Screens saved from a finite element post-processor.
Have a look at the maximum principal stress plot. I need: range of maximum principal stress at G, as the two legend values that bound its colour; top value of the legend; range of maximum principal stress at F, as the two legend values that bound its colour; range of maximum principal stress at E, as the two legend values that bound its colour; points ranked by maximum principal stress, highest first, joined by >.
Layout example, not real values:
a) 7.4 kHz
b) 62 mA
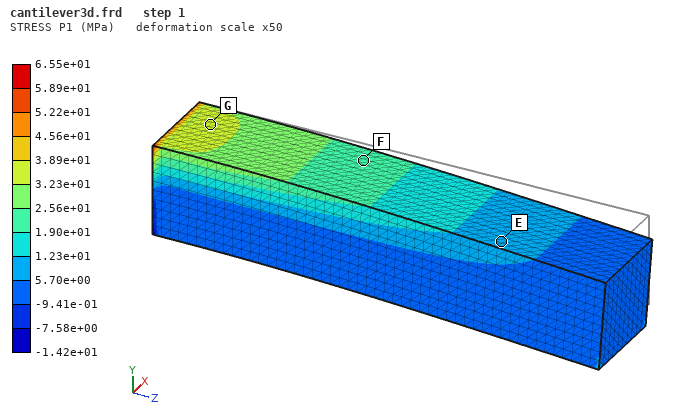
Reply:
a) 3.23e+01 to 3.89e+01 MPa
b) 6.55e+01 MPa
c) 1.90e+01 to 2.56e+01 MPa
d) 5.70e+00 to 1.23e+01 MPa
e) G > F > E
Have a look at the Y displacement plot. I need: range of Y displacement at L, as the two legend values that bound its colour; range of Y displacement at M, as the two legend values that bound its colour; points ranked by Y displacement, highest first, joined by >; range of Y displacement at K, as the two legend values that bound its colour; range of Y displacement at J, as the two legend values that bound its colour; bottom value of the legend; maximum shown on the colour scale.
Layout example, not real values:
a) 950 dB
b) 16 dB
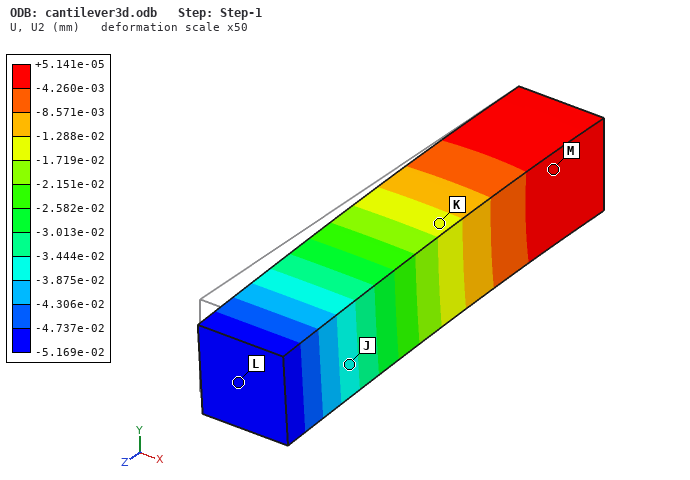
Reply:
a) -5.169e-02 to -4.737e-02 mm
b) -4.260e-03 to +5.141e-05 mm
c) M > K > J > L
d) -1.719e-02 to -1.288e-02 mm
e) -3.875e-02 to -3.444e-02 mm
f) -5.169e-02 mm
g) +5.141e-05 mm
